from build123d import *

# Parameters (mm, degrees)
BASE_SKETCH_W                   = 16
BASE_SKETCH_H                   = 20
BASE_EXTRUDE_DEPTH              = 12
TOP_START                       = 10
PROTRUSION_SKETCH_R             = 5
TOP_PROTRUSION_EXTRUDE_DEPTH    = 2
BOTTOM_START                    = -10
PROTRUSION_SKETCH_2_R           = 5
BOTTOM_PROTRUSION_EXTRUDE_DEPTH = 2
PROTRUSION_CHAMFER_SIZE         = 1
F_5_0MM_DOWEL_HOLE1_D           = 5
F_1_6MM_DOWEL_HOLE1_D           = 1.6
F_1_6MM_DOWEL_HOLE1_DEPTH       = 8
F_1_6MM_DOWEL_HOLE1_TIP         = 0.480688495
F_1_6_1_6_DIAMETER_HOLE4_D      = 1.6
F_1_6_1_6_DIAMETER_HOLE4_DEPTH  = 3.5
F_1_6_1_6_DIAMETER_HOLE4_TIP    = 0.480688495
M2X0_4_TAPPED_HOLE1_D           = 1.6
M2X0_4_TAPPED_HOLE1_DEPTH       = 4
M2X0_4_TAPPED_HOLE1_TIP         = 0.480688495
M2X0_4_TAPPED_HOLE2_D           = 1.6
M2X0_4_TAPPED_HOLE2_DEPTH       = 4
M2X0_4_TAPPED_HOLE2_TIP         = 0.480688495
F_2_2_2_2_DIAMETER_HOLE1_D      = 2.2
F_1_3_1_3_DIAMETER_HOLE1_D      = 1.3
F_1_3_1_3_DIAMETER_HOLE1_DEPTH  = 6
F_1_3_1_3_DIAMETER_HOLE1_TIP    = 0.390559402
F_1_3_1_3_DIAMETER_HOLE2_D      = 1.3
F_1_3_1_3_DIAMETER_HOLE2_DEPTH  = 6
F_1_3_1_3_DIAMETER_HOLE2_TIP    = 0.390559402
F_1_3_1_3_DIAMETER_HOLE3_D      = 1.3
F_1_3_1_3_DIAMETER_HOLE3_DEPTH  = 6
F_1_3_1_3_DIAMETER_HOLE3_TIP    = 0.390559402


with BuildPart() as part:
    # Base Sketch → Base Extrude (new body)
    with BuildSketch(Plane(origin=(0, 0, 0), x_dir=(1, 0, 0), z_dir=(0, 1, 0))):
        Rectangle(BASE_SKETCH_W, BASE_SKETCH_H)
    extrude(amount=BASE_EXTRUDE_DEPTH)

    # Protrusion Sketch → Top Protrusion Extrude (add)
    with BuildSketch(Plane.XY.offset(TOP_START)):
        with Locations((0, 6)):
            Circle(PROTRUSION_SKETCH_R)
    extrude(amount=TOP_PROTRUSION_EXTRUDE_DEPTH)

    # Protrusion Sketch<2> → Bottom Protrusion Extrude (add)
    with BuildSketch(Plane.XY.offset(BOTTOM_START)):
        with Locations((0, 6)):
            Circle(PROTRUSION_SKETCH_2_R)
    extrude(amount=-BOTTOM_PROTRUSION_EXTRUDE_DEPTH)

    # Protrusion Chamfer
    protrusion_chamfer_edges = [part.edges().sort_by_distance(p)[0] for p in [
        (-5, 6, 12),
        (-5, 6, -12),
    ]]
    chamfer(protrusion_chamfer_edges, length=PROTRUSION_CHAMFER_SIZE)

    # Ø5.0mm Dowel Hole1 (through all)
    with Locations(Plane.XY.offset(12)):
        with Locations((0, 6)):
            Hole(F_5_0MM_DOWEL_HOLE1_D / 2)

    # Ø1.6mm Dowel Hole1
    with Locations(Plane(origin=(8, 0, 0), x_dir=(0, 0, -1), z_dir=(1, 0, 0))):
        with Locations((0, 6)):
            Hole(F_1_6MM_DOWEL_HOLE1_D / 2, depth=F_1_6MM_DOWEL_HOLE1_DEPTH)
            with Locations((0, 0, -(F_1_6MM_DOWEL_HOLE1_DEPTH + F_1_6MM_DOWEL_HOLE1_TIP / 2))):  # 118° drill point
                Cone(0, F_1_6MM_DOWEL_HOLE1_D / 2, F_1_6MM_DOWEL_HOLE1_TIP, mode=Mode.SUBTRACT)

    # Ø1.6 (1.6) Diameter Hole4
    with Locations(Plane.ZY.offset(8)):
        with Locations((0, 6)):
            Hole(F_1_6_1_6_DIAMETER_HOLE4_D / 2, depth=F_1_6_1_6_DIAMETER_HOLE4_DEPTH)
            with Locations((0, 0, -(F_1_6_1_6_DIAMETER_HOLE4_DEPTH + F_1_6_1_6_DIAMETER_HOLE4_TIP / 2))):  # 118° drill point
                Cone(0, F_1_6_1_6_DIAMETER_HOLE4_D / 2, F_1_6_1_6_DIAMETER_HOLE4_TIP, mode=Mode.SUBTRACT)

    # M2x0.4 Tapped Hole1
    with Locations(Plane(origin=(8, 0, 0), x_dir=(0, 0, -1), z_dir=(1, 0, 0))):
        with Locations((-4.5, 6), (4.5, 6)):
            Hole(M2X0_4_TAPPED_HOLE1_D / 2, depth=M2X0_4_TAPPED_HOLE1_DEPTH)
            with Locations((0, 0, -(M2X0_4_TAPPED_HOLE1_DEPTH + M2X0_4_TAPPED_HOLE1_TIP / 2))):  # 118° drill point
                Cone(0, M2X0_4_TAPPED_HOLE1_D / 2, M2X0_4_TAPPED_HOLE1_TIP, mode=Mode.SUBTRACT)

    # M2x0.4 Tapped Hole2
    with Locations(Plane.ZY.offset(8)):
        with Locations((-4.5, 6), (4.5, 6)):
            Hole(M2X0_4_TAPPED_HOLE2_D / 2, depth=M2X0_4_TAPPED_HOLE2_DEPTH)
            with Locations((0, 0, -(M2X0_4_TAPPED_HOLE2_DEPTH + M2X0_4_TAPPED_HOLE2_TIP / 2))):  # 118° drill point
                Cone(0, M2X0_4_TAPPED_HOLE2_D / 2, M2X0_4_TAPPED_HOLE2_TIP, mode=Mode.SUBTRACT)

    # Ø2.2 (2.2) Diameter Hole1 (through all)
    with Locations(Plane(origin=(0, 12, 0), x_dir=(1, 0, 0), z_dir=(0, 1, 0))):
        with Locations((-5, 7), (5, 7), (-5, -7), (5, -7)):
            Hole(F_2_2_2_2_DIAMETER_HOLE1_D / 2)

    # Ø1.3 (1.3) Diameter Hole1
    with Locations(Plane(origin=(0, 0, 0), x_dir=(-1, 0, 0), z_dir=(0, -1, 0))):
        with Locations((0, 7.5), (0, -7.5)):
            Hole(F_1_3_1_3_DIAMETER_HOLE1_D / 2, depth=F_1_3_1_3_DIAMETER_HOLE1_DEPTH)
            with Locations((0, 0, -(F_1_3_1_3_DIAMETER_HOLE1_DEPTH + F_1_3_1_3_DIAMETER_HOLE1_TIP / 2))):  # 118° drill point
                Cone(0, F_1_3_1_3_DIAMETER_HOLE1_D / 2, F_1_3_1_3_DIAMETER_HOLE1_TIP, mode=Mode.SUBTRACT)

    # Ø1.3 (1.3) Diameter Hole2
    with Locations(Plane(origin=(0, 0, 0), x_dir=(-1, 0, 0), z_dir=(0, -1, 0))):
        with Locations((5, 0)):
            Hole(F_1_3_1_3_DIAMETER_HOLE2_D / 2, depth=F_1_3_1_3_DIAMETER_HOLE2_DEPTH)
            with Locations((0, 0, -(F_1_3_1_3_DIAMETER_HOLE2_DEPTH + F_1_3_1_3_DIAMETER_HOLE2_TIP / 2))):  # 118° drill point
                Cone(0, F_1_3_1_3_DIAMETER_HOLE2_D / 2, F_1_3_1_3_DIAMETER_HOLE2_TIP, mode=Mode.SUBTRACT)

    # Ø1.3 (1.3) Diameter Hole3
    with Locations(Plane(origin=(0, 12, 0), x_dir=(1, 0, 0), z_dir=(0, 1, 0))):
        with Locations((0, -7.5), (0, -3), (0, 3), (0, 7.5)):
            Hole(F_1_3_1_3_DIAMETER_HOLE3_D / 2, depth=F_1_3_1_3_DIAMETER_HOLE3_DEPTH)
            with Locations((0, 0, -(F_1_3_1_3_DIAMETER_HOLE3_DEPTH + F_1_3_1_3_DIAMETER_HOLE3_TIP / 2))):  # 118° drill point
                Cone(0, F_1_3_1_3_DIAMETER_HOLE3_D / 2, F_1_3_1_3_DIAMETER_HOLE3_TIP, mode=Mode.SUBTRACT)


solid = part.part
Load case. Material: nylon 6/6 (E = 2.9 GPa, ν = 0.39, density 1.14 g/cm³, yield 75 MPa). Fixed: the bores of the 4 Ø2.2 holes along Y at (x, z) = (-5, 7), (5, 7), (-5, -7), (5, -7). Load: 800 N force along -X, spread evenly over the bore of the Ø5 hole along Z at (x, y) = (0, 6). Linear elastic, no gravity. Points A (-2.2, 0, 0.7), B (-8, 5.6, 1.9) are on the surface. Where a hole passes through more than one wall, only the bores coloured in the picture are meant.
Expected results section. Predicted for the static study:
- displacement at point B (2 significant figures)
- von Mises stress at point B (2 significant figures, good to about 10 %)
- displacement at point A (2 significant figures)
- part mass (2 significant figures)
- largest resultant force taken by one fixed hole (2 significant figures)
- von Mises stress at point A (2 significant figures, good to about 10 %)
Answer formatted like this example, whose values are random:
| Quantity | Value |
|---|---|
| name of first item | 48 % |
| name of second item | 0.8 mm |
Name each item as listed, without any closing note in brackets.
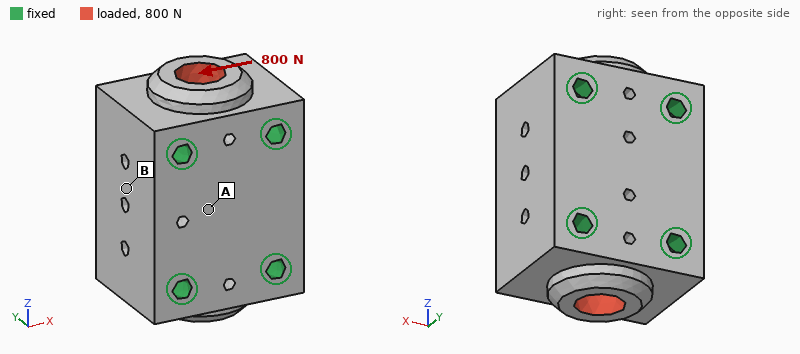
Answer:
| Quantity | Value |
|---|---|
| displacement at point B | 5.3 µm |
| von Mises stress at point B | 1.6 MPa |
| displacement at point A | 4.4 µm |
| part mass | 3.9 g |
| largest resultant force taken by one fixed hole | 200 N |
| von Mises stress at point A | 0.66 MPa |
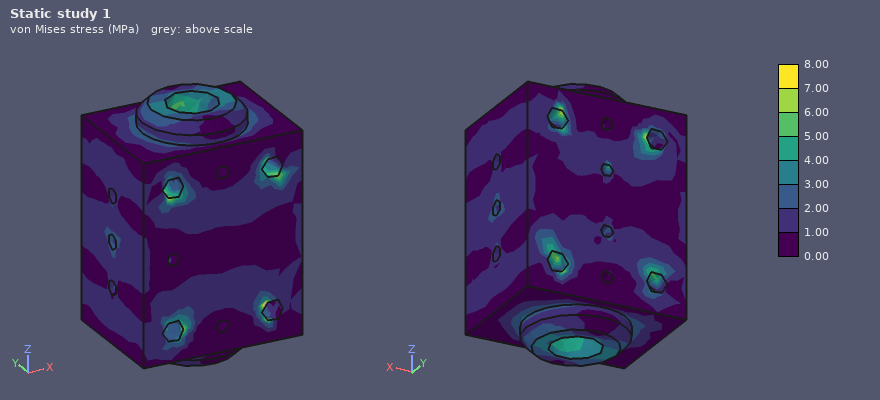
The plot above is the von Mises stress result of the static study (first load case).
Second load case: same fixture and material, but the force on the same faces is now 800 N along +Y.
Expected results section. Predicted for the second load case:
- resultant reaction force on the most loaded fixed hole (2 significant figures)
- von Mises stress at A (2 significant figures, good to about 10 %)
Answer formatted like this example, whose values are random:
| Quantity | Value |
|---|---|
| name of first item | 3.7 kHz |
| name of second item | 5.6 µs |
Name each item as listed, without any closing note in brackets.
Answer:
| Quantity | Value |
|---|---|
| resultant reaction force on the most loaded fixed hole | 200 N |
| von Mises stress at A | 2.2 MPa |
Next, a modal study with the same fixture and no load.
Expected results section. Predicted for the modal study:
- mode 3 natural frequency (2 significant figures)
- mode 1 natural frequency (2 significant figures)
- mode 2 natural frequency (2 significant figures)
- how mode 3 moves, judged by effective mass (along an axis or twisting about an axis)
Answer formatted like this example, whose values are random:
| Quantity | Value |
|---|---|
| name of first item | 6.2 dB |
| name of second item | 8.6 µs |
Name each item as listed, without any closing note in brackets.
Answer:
| Quantity | Value |
|---|---|
| mode 3 natural frequency | 33 kHz |
| mode 1 natural frequency | 30 kHz |
| mode 2 natural frequency | 31 kHz |
| how mode 3 moves, judged by effective mass | twisting about Z |
